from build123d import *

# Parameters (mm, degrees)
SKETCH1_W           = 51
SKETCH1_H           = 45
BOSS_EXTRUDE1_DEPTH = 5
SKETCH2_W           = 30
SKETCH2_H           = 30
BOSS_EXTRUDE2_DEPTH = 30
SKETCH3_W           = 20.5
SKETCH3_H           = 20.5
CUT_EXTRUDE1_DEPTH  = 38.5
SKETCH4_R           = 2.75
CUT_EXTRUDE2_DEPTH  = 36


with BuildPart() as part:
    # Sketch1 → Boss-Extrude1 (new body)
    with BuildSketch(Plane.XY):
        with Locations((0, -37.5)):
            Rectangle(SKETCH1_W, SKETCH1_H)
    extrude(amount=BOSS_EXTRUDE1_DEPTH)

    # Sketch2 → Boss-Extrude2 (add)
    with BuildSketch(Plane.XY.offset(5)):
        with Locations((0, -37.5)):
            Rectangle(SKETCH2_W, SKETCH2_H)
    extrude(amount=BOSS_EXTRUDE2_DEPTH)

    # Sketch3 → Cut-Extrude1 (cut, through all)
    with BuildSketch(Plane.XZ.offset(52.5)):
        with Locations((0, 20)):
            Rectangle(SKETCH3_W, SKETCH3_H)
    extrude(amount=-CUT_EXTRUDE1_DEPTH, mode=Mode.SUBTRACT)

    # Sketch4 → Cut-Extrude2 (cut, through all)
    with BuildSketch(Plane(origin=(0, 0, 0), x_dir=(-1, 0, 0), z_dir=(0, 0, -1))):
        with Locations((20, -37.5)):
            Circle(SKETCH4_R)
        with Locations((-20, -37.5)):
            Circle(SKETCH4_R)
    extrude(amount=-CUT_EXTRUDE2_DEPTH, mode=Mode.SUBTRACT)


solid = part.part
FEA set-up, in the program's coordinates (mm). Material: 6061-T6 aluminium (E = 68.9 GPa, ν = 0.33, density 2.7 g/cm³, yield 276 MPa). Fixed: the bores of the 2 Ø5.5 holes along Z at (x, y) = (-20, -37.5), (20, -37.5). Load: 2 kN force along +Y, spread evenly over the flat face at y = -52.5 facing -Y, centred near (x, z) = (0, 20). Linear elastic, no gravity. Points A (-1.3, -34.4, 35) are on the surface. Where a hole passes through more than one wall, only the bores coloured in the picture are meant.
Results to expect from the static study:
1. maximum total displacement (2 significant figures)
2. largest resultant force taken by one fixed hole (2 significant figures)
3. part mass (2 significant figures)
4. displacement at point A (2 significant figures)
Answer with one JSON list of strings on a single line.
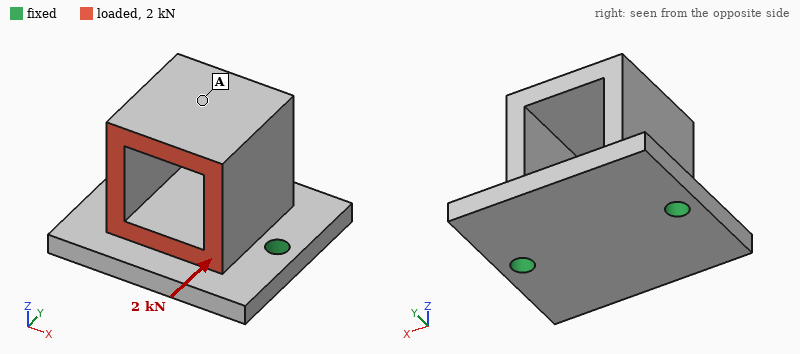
["0.13 mm", "1.0 kN", "69 g", "0.12 mm"]
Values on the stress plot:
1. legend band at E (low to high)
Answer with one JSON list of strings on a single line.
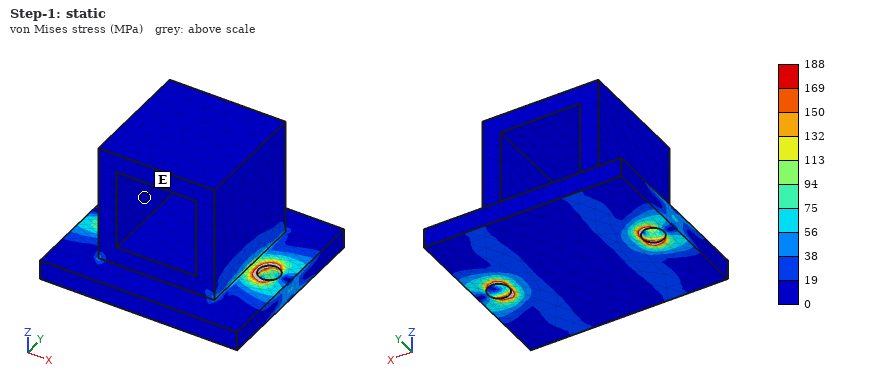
["0 to 19 MPa"]
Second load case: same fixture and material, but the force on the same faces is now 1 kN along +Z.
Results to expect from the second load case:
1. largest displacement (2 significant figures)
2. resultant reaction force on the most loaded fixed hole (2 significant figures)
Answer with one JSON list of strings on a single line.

["59 µm", "540 N"]
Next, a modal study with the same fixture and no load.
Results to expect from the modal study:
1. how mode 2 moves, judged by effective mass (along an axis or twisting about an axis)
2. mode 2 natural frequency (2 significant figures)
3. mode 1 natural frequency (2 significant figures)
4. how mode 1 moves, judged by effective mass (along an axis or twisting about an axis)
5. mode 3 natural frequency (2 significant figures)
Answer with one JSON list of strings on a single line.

["along X", "5200 Hz", "3300 Hz", "along Y", "9900 Hz"]
